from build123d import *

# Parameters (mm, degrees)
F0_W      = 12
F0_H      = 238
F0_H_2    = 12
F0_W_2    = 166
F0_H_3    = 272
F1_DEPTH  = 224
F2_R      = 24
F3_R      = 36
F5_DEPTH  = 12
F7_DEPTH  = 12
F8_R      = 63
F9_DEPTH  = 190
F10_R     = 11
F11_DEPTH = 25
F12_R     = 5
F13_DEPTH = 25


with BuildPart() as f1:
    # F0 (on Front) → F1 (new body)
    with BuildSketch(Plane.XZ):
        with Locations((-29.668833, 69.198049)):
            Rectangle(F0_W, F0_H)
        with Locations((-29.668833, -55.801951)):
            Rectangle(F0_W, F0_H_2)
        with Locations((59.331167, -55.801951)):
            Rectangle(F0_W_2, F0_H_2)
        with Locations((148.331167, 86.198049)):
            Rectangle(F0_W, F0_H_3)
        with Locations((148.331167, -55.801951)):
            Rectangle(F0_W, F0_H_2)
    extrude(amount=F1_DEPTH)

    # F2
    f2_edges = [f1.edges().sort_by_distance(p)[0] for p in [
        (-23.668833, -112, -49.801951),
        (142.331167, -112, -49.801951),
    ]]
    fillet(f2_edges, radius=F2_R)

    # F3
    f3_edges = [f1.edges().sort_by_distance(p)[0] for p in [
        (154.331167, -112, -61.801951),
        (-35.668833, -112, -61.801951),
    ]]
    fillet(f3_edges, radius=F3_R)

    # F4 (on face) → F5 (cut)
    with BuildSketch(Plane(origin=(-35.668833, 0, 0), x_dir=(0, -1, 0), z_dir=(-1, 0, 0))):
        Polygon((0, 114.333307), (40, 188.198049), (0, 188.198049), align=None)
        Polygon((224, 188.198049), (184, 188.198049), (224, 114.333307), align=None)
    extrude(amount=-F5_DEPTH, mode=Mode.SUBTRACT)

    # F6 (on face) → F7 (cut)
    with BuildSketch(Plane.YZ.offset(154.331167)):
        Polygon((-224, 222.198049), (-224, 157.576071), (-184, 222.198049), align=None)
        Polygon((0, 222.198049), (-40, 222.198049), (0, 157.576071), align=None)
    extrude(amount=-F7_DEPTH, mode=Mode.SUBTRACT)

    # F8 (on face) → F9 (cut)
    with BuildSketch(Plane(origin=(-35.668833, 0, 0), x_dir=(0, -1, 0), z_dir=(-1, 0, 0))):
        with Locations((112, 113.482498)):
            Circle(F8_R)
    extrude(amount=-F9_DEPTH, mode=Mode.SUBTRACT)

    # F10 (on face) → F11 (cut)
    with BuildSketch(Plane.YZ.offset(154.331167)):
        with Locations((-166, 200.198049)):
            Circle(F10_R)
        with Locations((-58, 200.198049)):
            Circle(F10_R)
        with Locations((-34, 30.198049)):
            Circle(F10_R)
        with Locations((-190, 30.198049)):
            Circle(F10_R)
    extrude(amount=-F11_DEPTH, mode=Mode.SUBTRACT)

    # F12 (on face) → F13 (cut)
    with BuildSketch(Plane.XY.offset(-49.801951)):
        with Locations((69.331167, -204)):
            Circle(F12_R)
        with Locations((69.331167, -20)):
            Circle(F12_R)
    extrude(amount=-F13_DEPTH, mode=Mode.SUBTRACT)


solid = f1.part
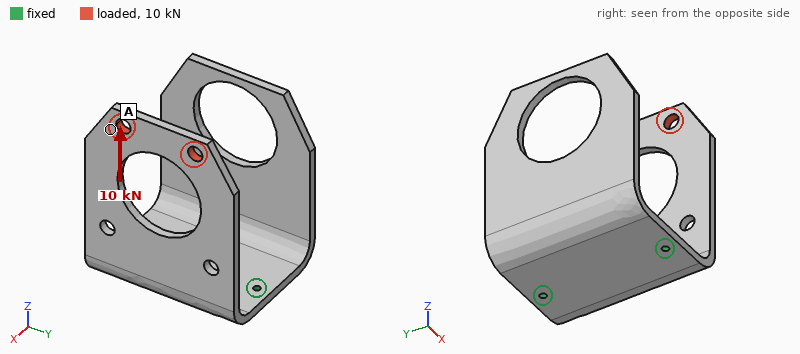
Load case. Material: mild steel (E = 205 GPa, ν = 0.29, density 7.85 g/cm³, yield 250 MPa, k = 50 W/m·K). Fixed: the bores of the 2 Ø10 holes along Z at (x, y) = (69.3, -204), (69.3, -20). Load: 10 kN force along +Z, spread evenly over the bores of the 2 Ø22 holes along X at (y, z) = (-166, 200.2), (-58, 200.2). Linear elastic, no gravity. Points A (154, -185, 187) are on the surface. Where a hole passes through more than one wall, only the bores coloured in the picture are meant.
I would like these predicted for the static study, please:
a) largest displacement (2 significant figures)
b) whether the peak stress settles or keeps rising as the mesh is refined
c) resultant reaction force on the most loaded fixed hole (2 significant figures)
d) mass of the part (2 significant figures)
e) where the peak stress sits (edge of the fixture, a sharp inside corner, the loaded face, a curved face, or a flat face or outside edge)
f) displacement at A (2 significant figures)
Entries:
1.8 mm
keeps rising
5.0 kN
11 kg
edge of the fixture
1.6 mm
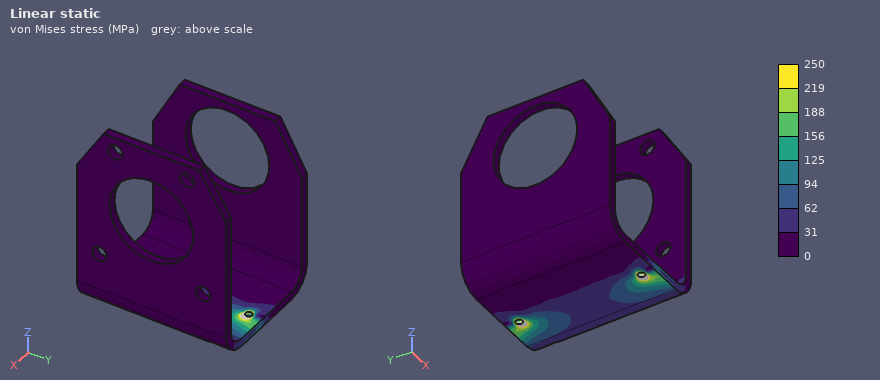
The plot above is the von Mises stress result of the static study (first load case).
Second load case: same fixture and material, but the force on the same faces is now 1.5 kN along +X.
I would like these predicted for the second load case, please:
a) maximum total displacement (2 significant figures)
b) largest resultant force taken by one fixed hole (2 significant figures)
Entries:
3.1 mm
770 N
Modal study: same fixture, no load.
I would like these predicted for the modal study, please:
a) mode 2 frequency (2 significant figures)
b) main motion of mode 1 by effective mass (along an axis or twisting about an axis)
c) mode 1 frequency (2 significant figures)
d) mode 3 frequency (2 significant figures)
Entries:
140 Hz
along X
100 Hz
270 Hz
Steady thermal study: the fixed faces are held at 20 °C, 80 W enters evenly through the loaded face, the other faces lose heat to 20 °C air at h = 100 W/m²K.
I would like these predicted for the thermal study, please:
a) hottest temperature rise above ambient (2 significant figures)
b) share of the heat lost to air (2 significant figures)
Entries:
42 K
100 %
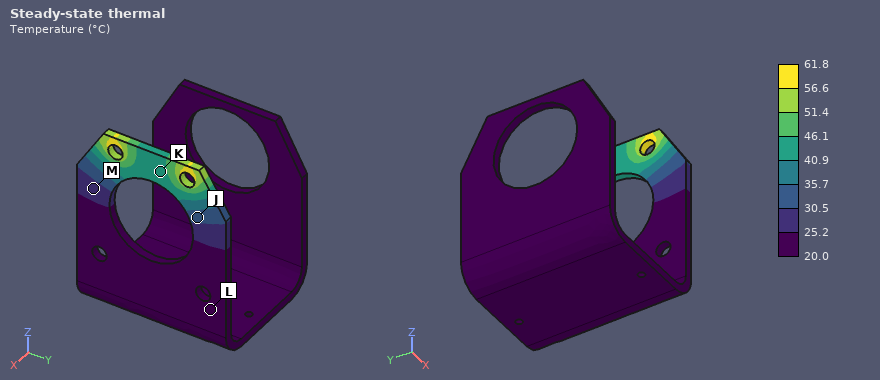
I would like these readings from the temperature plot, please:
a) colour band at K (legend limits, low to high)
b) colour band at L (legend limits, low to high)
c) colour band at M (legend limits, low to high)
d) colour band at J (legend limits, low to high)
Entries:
40.9 to 46.1 °C
20.0 to 25.2 °C
25.2 to 30.5 °C
30.5 to 35.7 °C
